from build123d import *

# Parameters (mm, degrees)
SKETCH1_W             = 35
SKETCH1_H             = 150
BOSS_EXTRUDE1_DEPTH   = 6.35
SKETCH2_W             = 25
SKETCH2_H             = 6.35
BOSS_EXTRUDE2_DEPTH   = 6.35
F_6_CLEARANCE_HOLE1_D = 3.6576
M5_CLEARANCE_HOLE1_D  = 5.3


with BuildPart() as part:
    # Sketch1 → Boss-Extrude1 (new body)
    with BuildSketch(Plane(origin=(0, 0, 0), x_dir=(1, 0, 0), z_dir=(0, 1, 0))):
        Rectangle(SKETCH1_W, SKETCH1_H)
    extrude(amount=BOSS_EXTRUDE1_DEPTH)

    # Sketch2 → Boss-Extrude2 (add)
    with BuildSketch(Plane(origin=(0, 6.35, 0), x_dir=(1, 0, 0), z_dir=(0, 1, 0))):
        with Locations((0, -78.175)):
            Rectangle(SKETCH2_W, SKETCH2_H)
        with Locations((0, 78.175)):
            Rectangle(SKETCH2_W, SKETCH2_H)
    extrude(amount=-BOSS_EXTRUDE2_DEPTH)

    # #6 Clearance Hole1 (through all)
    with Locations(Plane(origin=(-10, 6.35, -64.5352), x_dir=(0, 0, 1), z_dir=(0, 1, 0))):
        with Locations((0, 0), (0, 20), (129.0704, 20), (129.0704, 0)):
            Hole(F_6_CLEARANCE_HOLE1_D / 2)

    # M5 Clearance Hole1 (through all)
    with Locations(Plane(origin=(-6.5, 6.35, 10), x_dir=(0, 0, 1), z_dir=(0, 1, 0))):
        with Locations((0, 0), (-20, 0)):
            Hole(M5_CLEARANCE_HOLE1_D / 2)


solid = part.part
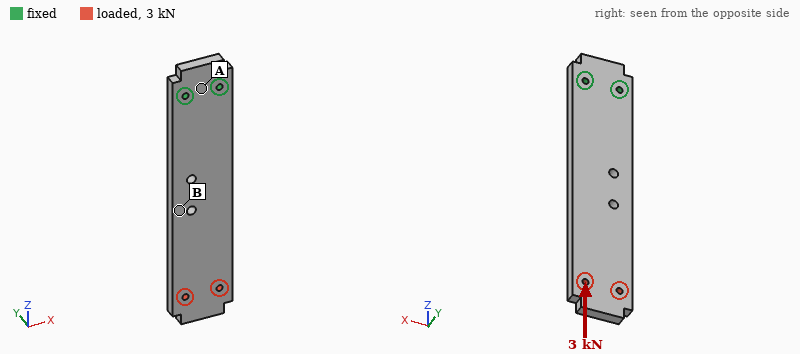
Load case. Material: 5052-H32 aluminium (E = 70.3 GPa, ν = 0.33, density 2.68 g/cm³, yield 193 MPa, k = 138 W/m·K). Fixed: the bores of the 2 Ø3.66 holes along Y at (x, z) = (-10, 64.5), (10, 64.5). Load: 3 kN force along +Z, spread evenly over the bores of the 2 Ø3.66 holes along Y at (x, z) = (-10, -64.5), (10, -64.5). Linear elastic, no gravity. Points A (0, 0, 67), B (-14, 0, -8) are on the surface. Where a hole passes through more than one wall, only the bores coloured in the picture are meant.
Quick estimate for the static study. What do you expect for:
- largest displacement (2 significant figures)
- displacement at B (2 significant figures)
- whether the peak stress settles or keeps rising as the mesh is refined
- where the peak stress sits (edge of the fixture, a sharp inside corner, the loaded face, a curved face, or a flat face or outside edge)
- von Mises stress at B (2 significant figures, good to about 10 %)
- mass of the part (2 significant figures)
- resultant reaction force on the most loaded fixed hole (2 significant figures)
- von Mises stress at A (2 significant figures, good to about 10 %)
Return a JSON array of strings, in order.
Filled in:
["28 µm", "15 µm", "keeps rising", "edge of the fixture", "16 MPa", "93 g", "1.5 kN", "5.1 MPa"]
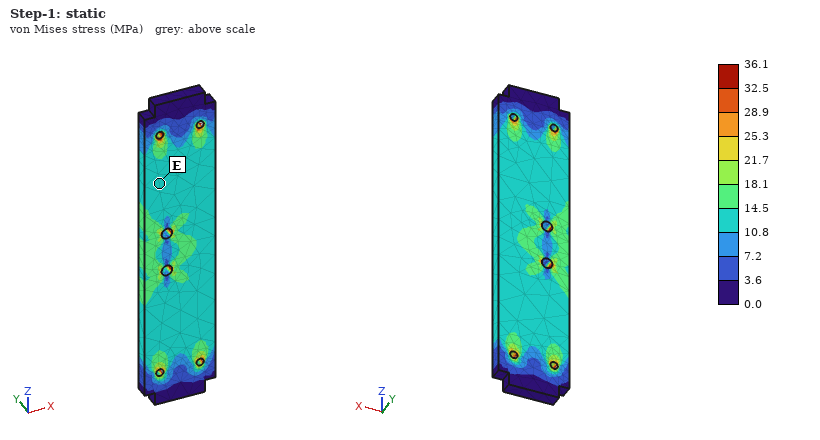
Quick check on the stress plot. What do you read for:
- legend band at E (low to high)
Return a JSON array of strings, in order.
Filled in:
["10.8 to 14.5 MPa"]
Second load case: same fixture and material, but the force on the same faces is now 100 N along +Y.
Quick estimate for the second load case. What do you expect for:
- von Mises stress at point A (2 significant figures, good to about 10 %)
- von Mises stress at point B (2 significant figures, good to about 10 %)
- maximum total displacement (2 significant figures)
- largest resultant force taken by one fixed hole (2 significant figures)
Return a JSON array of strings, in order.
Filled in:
["16 MPa", "28 MPa", "1.7 mm", "50 N"]
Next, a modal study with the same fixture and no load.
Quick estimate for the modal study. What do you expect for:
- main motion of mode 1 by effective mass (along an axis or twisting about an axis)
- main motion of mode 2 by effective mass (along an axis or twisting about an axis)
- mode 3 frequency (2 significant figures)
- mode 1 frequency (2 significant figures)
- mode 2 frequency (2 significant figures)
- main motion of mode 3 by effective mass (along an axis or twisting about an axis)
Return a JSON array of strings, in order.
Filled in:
["along Y", "along X", "1600 Hz", "250 Hz", "1300 Hz", "along Y"]
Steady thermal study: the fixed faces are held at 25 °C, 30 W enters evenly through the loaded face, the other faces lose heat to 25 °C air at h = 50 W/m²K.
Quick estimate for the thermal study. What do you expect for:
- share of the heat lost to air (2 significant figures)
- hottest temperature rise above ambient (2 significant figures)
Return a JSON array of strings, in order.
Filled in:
["65 %", "68 K"]
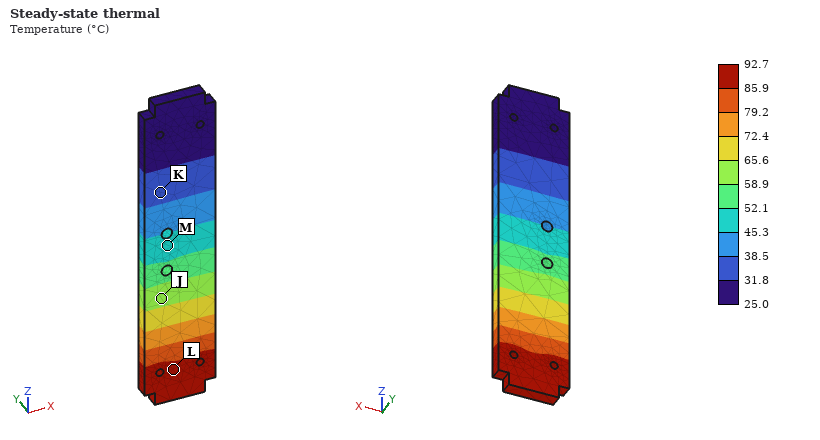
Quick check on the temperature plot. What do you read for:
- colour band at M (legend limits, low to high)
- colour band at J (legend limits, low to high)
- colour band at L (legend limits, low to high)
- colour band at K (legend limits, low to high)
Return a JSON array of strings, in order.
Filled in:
["45.3 to 52.1 °C", "58.9 to 65.6 °C", "85.9 to 92.7 °C", "31.8 to 38.5 °C"]
